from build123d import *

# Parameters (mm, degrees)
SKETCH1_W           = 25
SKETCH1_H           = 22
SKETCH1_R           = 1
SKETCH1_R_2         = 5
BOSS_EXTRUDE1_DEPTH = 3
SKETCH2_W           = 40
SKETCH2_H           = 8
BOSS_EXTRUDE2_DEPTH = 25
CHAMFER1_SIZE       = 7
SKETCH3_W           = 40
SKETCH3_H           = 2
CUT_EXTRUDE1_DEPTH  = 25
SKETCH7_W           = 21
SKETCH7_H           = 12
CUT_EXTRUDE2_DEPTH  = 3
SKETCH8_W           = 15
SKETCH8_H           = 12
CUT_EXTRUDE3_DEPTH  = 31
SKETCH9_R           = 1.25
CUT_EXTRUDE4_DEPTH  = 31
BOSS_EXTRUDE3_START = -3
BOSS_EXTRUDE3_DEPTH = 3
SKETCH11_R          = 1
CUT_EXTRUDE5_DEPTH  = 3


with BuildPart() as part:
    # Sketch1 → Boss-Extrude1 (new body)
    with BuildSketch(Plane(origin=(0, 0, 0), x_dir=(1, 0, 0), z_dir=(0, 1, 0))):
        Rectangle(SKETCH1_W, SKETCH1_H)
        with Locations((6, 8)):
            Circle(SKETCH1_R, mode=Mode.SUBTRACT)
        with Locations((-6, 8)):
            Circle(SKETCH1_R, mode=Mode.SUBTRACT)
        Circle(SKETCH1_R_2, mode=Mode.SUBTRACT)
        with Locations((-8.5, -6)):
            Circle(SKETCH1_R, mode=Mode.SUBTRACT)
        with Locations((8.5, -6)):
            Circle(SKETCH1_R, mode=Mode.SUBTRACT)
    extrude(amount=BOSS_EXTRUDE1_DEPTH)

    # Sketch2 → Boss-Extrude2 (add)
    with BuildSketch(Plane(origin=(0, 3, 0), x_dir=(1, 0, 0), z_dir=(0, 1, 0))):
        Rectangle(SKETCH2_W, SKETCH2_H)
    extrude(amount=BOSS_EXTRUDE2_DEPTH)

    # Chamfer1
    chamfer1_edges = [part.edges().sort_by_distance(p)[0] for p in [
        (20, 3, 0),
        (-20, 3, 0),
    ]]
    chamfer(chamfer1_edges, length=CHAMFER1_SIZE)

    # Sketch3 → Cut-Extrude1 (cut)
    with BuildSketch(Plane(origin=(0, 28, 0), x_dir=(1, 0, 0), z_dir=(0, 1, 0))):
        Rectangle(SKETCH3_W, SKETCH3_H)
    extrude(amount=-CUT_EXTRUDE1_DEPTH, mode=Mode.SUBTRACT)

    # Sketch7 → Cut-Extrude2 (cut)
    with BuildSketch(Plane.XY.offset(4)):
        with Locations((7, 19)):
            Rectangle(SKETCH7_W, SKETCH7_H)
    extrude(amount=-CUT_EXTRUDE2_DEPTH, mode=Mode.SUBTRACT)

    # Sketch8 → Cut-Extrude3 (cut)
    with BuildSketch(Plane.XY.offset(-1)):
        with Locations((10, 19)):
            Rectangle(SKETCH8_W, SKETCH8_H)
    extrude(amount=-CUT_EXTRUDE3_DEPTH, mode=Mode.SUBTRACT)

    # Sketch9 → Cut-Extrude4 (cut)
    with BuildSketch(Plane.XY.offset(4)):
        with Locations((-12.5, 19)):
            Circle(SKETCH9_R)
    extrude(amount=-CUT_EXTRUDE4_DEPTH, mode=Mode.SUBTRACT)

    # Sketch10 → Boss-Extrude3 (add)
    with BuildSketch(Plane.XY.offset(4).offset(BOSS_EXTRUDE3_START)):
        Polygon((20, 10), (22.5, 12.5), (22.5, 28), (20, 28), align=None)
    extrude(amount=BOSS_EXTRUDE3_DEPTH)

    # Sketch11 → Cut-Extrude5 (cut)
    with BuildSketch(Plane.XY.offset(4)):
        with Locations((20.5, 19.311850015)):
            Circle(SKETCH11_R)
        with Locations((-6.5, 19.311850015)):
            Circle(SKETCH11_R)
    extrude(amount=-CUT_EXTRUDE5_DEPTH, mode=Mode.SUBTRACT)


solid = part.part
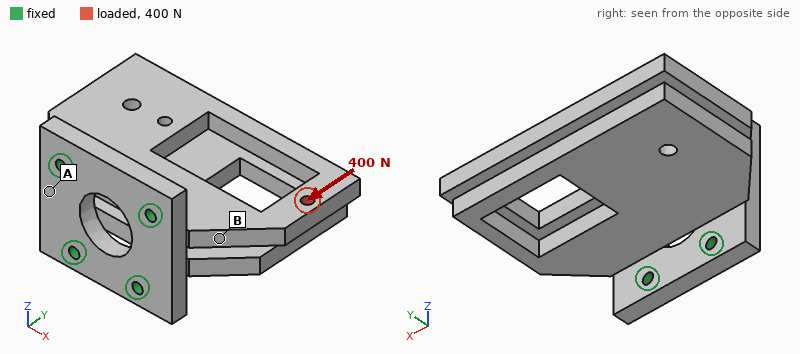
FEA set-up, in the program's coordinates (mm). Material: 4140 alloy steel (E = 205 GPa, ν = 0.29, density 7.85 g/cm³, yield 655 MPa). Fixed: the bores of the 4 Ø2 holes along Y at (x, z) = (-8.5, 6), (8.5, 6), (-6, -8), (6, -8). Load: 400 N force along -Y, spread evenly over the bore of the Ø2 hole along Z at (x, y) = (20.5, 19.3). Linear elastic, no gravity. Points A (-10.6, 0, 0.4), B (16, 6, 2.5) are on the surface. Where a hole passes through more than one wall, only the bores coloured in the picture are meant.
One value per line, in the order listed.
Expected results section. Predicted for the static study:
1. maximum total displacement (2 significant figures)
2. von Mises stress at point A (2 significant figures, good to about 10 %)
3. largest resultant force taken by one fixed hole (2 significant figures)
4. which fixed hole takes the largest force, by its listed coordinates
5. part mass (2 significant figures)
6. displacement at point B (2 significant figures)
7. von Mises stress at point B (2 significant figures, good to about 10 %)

15 µm
13 MPa
540 N
(8.5, 6)
46 g
6.0 µm
60 MPa
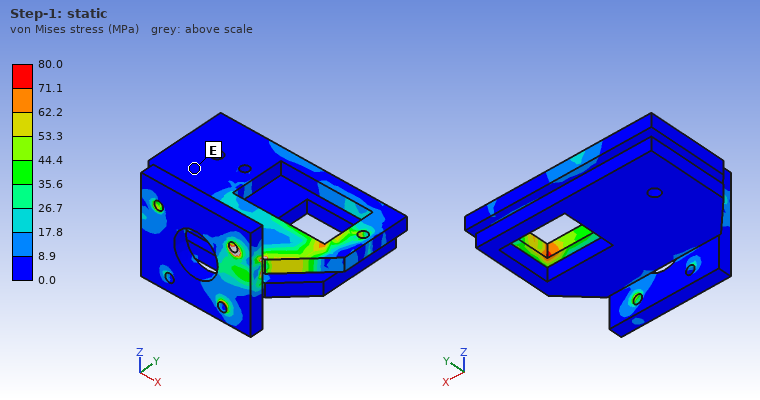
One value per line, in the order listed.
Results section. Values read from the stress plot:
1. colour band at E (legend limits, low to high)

0.0 to 8.9 MPa
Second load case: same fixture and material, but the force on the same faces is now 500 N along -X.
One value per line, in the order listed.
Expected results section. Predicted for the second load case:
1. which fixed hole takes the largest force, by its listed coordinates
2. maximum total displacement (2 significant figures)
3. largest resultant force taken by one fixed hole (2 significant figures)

(8.5, 6)
20 µm
480 N
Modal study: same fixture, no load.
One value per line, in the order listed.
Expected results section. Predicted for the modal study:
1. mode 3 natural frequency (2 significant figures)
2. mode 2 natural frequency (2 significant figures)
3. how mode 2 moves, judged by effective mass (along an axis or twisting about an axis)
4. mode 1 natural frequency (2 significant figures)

4000 Hz
2900 Hz
along Z
2700 Hz
